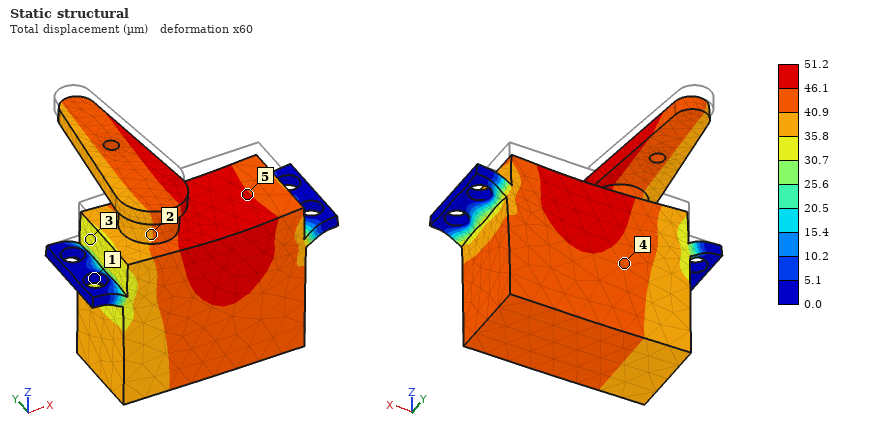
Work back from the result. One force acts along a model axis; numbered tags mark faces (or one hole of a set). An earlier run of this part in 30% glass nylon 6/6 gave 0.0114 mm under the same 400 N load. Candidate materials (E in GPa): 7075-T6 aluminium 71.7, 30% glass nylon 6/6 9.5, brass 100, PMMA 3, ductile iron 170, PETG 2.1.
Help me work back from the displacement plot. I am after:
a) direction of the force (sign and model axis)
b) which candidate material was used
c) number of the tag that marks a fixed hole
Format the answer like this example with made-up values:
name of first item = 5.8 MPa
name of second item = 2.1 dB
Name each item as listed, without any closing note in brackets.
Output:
direction of the force = -Z
which candidate material was used = PETG
number of the tag that marks a fixed hole = 1
